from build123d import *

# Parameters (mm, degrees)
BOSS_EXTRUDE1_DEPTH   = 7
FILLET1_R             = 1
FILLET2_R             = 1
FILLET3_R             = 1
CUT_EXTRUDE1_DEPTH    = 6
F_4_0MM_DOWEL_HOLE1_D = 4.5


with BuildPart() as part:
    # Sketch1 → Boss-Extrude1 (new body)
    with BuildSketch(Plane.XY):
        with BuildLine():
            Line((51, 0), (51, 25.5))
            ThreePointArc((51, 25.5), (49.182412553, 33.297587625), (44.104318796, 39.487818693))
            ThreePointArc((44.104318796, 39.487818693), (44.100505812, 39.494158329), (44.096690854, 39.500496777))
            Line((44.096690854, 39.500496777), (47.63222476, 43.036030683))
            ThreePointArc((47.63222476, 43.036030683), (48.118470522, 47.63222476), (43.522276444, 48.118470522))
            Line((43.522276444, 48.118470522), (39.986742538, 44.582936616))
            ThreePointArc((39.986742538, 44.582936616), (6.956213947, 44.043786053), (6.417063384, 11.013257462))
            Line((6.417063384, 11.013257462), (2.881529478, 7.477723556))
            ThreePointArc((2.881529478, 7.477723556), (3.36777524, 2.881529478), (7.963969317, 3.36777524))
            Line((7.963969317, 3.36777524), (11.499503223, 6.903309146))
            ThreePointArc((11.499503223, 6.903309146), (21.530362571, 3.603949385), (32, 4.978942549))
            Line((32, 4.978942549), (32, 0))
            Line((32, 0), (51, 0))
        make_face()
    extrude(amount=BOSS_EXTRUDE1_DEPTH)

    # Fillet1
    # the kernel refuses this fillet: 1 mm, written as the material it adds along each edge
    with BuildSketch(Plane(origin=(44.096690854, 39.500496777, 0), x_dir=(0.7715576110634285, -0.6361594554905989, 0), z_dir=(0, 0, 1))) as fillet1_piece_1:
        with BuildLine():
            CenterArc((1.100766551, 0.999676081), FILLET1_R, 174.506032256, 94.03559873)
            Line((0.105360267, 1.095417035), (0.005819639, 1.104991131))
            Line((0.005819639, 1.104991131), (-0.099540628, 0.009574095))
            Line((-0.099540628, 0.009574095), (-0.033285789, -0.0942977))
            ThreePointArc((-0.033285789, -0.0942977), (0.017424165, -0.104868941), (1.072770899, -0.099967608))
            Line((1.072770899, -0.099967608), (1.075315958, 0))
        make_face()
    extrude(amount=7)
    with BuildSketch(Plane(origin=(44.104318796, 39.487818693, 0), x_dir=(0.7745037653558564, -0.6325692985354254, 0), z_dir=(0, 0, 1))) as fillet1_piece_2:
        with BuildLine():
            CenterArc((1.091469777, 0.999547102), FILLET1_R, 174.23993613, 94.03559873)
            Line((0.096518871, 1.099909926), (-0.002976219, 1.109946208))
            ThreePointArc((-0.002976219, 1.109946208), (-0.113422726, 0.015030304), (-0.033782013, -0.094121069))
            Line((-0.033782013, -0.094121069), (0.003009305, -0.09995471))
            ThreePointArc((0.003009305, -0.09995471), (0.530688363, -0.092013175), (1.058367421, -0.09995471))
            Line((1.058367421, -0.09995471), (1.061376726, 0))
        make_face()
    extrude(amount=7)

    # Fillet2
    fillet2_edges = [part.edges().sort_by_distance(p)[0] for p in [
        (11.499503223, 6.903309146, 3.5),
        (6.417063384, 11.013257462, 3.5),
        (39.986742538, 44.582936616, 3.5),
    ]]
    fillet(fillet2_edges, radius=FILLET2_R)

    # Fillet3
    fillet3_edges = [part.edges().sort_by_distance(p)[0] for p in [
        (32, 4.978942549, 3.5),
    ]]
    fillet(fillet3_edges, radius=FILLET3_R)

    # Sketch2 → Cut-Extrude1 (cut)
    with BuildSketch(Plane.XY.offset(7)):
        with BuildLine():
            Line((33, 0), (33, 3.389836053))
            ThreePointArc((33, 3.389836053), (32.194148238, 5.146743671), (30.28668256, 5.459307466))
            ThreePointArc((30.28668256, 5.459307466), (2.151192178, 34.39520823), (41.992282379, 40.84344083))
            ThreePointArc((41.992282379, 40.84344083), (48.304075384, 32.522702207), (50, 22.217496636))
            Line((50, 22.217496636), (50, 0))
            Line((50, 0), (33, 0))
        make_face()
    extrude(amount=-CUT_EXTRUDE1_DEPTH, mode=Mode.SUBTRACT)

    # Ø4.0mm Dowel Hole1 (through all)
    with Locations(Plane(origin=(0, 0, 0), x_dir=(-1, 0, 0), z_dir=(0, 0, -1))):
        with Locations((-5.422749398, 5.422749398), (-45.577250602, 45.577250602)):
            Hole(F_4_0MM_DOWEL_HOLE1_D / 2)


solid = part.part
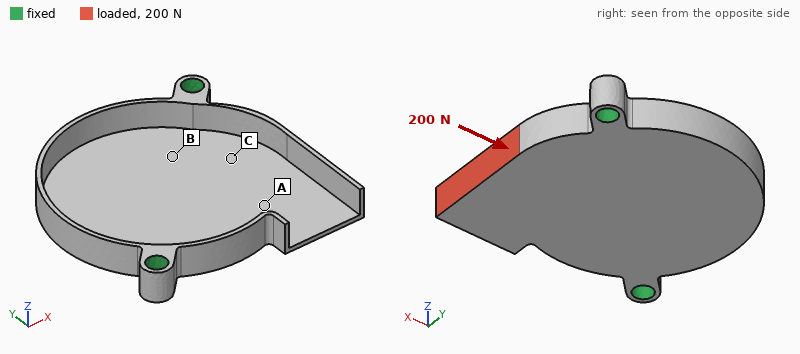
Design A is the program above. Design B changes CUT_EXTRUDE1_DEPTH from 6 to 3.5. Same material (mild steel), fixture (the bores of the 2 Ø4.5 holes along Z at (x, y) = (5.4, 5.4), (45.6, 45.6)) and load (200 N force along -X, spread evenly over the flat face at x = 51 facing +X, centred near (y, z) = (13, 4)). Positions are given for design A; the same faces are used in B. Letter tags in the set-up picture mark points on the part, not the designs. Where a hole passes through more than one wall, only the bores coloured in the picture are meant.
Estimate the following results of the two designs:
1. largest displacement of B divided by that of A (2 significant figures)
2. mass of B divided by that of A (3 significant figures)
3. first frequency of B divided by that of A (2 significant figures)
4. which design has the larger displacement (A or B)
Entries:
0.068
2.40
1.3
A
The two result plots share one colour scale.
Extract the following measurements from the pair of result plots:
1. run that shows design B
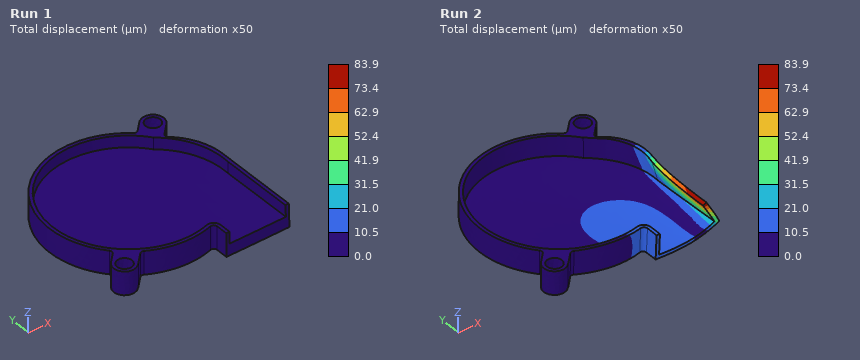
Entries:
Run 1
